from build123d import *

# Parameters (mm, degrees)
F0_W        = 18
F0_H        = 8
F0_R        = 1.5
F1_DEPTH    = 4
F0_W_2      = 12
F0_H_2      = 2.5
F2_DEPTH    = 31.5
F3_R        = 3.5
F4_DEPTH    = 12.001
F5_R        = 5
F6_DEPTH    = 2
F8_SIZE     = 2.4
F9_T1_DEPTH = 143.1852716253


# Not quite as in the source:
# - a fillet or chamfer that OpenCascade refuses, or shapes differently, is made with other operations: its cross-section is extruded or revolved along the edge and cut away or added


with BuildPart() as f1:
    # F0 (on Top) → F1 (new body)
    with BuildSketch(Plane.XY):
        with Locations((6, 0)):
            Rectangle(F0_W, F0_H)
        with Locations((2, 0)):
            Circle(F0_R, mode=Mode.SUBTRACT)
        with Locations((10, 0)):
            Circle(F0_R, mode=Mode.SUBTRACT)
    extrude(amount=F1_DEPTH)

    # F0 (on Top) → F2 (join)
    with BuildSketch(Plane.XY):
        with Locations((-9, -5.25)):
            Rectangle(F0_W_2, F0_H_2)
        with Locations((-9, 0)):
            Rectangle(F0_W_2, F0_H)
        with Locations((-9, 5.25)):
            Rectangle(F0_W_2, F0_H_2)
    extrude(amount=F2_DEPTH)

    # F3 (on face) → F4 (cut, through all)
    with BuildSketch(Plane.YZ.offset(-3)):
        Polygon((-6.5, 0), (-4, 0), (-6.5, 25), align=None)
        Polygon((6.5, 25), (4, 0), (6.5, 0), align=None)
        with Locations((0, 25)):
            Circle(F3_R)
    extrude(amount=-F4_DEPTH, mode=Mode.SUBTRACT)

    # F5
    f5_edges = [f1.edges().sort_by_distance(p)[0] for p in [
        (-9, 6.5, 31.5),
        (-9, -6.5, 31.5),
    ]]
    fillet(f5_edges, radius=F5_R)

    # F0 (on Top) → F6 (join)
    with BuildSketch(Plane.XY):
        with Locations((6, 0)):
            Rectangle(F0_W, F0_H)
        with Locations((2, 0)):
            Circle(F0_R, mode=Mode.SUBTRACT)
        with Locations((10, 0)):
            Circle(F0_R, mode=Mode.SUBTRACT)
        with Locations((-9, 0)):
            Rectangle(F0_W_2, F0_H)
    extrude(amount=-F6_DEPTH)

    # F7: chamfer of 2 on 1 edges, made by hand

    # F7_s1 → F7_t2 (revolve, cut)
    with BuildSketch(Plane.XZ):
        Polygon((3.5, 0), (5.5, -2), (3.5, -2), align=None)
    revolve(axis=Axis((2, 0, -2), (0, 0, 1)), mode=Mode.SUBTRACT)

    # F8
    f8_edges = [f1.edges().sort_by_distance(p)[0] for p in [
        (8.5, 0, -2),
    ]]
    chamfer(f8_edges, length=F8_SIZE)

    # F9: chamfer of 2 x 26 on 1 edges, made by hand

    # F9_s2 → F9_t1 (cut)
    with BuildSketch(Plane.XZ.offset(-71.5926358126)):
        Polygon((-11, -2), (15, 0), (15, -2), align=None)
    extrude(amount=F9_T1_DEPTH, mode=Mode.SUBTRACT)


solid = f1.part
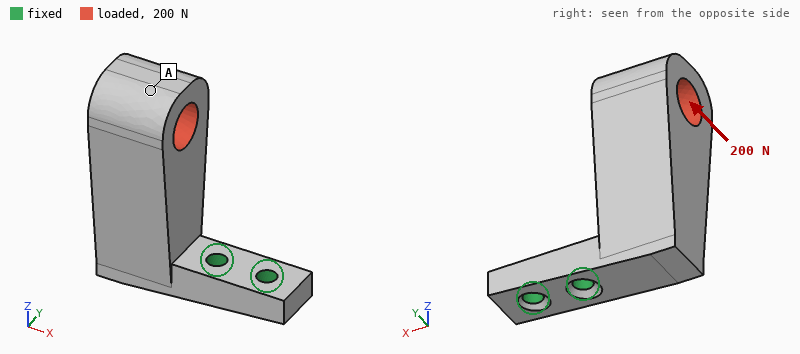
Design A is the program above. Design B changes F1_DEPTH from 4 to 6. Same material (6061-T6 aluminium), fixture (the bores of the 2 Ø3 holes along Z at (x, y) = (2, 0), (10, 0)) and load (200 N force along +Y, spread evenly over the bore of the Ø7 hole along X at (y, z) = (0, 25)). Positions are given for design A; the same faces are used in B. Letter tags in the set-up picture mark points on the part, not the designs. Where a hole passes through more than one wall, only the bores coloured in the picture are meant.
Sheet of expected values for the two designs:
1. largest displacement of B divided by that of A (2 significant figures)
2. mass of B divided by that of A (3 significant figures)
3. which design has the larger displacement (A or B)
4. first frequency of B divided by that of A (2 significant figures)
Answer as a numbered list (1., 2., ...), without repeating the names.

1. 0.54
2. 1.06
3. A
4. 1.5
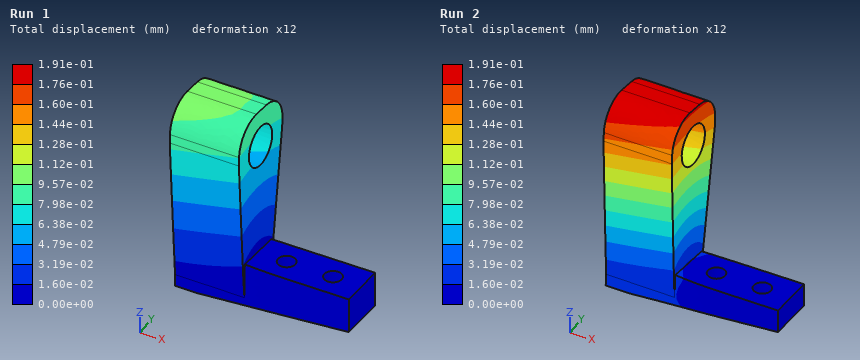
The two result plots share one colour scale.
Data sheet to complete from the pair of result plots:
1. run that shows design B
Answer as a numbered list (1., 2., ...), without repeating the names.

1. Run 1
